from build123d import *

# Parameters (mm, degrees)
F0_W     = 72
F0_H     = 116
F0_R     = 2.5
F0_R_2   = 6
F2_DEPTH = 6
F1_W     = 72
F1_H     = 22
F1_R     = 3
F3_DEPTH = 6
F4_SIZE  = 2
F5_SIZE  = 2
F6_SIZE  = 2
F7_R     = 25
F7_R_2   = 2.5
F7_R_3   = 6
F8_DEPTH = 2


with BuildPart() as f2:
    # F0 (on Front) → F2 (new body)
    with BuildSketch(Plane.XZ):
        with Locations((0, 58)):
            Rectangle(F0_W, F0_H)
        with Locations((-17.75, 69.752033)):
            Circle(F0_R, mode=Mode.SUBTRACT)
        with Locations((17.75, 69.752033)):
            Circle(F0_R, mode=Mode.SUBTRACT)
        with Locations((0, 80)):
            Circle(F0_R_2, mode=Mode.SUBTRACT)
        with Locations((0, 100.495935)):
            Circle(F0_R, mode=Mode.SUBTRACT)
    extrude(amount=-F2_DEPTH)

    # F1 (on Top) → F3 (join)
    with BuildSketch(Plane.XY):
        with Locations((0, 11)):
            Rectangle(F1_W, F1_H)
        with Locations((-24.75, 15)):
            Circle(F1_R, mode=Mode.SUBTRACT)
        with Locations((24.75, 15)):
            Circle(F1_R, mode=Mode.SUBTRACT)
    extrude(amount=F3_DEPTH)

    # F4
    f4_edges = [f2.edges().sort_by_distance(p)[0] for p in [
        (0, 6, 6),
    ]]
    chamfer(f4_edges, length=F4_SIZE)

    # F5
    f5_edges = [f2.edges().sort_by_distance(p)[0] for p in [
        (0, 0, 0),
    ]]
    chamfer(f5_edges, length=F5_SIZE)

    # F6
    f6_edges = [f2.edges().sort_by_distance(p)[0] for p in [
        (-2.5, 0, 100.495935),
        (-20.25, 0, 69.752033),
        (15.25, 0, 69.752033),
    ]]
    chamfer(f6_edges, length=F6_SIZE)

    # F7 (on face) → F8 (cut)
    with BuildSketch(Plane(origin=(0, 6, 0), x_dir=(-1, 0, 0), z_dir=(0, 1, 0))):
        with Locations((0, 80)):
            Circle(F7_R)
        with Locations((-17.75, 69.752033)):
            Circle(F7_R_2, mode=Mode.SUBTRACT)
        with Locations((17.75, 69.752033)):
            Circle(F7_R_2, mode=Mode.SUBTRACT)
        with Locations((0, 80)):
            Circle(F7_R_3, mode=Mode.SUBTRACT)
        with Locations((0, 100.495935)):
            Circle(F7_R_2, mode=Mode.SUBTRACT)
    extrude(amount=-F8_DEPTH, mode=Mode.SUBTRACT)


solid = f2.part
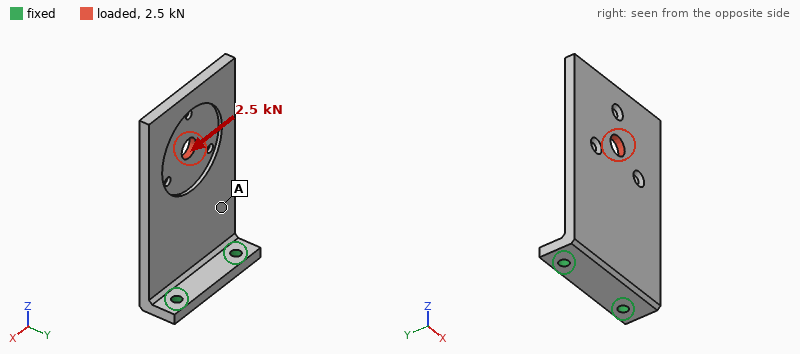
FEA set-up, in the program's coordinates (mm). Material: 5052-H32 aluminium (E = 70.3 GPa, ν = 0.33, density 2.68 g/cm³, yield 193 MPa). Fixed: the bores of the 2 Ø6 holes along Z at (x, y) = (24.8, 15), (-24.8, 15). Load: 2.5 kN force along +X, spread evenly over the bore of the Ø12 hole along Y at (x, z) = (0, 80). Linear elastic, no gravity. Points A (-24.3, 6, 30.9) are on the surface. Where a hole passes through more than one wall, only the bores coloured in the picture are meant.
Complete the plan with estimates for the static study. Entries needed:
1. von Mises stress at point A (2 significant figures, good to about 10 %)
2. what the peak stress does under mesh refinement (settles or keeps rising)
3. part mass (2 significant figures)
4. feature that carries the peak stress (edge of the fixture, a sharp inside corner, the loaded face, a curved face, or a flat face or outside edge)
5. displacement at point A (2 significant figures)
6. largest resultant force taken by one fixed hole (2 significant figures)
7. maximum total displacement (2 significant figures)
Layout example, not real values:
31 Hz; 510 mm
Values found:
31 MPa; keeps rising; 140 g; edge of the fixture; 0.10 mm; 3.9 kN; 0.31 mm
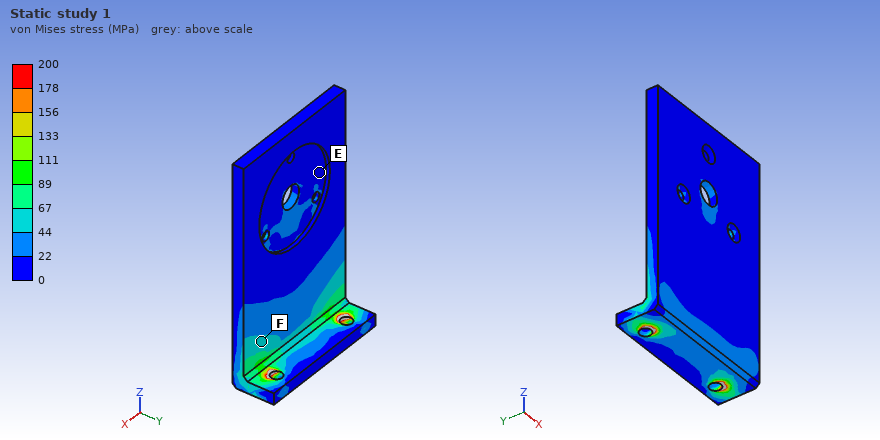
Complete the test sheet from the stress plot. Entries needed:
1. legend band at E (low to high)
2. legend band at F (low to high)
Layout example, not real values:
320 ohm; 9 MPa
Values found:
0 to 22 MPa; 44 to 67 MPa
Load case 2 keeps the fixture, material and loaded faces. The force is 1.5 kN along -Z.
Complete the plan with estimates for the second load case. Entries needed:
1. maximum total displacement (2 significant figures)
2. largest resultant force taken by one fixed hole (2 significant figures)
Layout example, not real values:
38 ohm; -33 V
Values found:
0.27 mm; 750 N
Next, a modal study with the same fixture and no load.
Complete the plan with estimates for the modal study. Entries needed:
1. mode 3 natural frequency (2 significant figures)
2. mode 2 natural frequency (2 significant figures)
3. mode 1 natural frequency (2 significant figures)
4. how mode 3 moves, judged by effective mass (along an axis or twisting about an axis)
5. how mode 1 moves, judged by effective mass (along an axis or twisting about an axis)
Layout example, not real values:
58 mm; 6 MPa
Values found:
1900 Hz; 1200 Hz; 360 Hz; along Y; along Y
